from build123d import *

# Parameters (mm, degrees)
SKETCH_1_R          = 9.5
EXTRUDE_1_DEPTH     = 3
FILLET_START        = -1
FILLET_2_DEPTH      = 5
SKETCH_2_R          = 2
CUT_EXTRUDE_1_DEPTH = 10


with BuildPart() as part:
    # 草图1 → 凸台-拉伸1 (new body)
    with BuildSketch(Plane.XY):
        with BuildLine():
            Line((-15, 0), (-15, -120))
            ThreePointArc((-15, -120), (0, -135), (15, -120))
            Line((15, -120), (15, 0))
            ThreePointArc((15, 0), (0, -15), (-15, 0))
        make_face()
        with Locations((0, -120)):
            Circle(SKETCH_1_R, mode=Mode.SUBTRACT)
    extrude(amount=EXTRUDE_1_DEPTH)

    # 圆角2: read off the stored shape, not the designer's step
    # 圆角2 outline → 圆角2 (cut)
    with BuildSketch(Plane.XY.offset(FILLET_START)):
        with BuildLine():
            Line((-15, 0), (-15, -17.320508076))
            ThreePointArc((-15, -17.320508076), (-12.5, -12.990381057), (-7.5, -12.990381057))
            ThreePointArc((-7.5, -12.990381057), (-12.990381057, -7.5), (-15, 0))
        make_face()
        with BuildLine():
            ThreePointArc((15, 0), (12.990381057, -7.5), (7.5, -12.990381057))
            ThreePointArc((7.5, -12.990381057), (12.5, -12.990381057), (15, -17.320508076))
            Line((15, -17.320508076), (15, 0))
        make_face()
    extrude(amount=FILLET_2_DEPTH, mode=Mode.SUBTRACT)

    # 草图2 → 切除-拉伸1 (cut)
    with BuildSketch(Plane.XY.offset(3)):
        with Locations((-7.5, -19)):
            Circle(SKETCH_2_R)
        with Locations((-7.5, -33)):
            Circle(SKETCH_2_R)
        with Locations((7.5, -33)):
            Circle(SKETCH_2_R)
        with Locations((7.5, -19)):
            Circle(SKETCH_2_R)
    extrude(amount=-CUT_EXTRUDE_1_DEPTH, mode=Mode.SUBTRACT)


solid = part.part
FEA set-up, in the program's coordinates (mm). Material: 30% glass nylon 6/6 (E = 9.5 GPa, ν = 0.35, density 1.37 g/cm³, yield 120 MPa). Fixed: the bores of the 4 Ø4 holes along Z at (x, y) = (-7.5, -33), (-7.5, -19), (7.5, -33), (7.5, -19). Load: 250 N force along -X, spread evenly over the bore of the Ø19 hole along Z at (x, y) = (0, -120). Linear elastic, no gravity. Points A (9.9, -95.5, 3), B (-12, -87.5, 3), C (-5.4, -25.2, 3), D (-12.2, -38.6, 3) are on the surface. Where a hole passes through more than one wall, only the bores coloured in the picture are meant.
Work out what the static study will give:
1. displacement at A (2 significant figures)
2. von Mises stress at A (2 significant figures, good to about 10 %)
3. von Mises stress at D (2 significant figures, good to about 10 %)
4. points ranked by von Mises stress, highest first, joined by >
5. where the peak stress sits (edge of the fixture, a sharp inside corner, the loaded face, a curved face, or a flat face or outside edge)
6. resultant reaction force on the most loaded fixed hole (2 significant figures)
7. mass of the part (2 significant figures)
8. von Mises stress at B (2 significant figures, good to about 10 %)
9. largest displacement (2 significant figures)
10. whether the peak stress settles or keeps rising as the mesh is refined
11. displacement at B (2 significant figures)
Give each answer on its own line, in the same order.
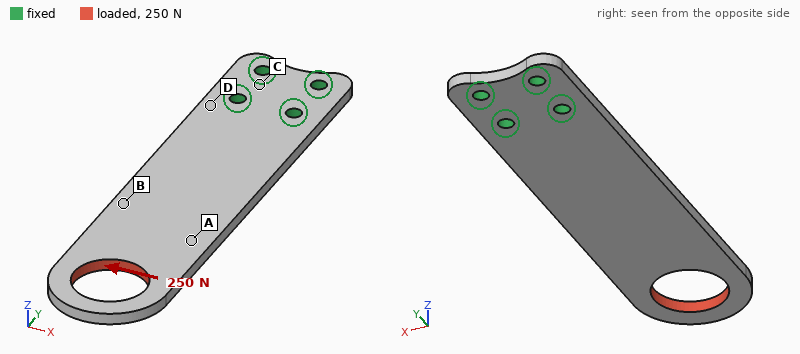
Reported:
0.63 mm
9.4 MPa
33 MPa
D > B > A > C
edge of the fixture
990 N
13 g
15 MPa
1.3 mm
keeps rising
0.52 mm
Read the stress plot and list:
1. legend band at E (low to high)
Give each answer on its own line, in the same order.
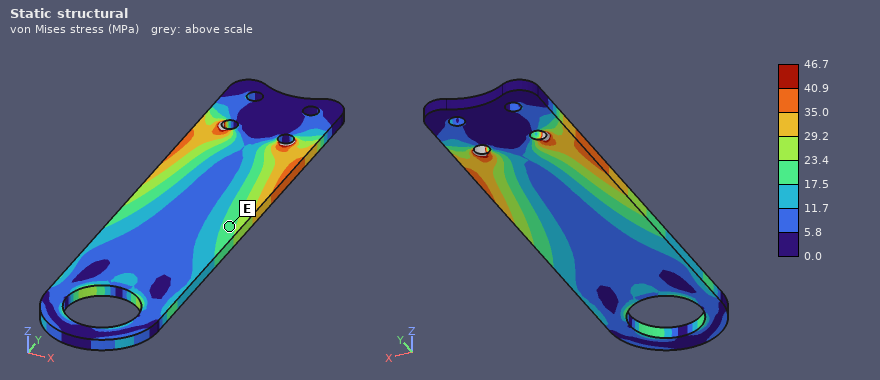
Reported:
17.5 to 23.4 MPa
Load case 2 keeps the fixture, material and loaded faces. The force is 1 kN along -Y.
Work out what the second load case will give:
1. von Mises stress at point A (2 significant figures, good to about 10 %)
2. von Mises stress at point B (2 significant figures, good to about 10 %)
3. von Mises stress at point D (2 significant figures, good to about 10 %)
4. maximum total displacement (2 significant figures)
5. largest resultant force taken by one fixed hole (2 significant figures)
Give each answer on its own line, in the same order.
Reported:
12 MPa
12 MPa
9.6 MPa
0.19 mm
440 N
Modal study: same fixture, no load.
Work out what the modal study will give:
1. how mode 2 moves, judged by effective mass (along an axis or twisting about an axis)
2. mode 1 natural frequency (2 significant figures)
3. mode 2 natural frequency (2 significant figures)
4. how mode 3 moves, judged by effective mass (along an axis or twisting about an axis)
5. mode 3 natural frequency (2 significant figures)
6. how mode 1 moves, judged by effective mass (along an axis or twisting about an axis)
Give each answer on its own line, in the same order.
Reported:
along Z
160 Hz
860 Hz
twisting about Y
900 Hz
along Z
